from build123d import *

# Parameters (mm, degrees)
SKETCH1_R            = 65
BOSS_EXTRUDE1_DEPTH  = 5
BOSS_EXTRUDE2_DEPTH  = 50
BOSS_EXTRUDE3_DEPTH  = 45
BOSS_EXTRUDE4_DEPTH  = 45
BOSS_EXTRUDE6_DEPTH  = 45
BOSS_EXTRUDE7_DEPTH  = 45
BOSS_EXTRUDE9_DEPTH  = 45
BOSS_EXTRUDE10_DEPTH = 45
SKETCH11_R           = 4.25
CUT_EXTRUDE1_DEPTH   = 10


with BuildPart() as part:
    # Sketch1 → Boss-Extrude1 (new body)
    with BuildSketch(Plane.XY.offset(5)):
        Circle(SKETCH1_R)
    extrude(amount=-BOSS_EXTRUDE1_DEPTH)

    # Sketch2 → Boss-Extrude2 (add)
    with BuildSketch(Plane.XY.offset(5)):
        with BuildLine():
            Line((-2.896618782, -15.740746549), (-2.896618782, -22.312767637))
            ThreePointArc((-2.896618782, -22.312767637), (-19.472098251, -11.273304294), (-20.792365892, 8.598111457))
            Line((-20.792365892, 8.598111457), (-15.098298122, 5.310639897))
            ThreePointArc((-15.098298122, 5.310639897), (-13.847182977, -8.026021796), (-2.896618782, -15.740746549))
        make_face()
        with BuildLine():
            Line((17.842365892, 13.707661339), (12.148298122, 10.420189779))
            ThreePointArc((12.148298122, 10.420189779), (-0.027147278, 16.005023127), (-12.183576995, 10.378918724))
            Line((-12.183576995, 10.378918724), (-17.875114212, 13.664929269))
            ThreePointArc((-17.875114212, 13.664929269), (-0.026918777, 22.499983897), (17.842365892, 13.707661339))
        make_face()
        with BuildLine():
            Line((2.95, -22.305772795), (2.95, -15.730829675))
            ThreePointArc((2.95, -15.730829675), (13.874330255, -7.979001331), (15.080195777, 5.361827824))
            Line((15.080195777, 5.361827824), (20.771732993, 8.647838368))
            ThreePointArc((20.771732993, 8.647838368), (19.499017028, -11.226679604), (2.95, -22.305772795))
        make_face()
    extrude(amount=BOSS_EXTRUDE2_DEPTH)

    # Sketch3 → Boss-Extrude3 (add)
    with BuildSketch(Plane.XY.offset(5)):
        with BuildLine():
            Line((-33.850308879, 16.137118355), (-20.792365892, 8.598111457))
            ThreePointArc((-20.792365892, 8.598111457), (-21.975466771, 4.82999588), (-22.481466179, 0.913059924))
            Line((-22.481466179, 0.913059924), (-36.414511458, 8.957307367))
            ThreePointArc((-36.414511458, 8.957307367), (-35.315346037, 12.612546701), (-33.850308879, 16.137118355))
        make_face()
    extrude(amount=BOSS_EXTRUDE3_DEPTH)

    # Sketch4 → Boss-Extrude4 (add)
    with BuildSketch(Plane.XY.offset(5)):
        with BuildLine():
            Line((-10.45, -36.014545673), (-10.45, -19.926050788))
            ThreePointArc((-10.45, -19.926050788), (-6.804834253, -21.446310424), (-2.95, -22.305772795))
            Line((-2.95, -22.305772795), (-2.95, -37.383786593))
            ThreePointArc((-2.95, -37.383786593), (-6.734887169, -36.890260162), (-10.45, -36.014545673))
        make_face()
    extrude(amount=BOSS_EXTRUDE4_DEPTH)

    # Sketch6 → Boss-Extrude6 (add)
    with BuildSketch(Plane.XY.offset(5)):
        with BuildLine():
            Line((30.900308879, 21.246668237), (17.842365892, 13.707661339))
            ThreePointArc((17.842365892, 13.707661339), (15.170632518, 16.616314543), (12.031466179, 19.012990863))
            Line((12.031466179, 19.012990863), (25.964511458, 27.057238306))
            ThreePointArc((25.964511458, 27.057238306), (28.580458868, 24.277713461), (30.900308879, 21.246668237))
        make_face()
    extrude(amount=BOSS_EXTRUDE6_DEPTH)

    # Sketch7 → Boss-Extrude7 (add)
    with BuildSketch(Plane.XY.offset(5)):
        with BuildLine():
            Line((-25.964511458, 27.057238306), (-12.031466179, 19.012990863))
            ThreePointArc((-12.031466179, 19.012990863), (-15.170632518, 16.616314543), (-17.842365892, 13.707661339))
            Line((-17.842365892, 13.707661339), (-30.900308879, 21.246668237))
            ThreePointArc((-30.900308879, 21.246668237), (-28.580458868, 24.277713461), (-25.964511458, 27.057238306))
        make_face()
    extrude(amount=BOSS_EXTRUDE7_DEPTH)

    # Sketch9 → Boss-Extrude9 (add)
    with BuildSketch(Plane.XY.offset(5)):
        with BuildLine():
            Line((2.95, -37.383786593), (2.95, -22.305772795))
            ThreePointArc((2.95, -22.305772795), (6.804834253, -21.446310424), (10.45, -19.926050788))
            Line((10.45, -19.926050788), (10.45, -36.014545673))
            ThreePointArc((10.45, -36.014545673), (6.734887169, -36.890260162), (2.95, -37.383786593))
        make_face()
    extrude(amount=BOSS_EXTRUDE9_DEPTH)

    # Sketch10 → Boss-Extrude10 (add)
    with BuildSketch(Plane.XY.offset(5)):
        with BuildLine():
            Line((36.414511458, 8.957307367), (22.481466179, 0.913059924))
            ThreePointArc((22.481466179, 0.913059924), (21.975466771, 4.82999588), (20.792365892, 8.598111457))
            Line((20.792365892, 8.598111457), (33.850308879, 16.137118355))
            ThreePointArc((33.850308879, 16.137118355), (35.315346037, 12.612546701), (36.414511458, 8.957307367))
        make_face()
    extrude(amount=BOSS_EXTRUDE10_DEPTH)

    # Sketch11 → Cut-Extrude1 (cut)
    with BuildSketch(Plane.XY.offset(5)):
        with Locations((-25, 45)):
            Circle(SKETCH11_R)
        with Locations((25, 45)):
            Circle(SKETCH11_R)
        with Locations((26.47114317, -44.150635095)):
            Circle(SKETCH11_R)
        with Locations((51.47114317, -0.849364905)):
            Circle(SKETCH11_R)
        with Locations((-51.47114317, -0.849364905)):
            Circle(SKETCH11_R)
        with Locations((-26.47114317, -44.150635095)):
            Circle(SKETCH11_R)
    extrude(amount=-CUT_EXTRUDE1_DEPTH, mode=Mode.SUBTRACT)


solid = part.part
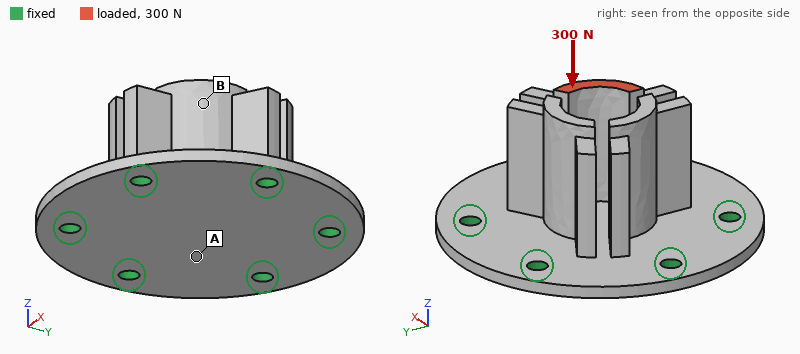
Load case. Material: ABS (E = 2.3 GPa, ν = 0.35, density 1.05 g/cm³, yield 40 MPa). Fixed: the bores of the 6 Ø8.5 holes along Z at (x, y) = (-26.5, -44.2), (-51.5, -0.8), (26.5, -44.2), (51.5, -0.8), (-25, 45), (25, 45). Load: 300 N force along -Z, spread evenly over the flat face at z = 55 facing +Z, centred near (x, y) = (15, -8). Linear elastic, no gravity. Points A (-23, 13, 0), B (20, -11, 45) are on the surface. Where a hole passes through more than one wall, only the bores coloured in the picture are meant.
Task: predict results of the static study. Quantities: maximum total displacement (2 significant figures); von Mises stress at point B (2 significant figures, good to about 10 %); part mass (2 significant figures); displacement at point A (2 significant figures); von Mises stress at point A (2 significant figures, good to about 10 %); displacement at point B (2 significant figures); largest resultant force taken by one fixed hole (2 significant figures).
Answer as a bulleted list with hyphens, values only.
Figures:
- 0.37 mm
- 1.2 MPa
- 140 g
- 0.084 mm
- 2.4 MPa
- 0.27 mm
- 84 N
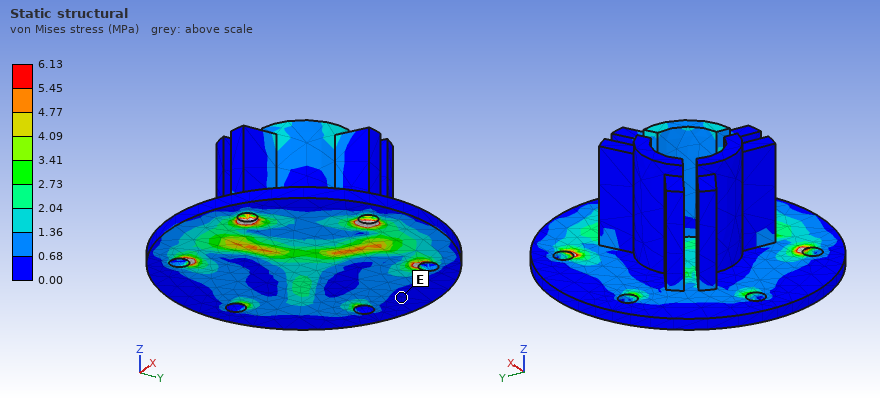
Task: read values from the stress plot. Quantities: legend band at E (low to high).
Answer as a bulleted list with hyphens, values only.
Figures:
- 0.00 to 0.68 MPa
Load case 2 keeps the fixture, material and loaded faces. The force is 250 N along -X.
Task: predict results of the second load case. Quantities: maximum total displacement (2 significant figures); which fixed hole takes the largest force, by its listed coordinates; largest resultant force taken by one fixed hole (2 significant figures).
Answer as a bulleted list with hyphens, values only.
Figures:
- 2.2 mm
- (51.5, -0.8)
- 170 N
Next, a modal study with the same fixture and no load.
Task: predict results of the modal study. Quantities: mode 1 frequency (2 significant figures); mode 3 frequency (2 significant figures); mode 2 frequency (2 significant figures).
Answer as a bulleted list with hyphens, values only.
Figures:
- 490 Hz
- 790 Hz
- 790 Hz
